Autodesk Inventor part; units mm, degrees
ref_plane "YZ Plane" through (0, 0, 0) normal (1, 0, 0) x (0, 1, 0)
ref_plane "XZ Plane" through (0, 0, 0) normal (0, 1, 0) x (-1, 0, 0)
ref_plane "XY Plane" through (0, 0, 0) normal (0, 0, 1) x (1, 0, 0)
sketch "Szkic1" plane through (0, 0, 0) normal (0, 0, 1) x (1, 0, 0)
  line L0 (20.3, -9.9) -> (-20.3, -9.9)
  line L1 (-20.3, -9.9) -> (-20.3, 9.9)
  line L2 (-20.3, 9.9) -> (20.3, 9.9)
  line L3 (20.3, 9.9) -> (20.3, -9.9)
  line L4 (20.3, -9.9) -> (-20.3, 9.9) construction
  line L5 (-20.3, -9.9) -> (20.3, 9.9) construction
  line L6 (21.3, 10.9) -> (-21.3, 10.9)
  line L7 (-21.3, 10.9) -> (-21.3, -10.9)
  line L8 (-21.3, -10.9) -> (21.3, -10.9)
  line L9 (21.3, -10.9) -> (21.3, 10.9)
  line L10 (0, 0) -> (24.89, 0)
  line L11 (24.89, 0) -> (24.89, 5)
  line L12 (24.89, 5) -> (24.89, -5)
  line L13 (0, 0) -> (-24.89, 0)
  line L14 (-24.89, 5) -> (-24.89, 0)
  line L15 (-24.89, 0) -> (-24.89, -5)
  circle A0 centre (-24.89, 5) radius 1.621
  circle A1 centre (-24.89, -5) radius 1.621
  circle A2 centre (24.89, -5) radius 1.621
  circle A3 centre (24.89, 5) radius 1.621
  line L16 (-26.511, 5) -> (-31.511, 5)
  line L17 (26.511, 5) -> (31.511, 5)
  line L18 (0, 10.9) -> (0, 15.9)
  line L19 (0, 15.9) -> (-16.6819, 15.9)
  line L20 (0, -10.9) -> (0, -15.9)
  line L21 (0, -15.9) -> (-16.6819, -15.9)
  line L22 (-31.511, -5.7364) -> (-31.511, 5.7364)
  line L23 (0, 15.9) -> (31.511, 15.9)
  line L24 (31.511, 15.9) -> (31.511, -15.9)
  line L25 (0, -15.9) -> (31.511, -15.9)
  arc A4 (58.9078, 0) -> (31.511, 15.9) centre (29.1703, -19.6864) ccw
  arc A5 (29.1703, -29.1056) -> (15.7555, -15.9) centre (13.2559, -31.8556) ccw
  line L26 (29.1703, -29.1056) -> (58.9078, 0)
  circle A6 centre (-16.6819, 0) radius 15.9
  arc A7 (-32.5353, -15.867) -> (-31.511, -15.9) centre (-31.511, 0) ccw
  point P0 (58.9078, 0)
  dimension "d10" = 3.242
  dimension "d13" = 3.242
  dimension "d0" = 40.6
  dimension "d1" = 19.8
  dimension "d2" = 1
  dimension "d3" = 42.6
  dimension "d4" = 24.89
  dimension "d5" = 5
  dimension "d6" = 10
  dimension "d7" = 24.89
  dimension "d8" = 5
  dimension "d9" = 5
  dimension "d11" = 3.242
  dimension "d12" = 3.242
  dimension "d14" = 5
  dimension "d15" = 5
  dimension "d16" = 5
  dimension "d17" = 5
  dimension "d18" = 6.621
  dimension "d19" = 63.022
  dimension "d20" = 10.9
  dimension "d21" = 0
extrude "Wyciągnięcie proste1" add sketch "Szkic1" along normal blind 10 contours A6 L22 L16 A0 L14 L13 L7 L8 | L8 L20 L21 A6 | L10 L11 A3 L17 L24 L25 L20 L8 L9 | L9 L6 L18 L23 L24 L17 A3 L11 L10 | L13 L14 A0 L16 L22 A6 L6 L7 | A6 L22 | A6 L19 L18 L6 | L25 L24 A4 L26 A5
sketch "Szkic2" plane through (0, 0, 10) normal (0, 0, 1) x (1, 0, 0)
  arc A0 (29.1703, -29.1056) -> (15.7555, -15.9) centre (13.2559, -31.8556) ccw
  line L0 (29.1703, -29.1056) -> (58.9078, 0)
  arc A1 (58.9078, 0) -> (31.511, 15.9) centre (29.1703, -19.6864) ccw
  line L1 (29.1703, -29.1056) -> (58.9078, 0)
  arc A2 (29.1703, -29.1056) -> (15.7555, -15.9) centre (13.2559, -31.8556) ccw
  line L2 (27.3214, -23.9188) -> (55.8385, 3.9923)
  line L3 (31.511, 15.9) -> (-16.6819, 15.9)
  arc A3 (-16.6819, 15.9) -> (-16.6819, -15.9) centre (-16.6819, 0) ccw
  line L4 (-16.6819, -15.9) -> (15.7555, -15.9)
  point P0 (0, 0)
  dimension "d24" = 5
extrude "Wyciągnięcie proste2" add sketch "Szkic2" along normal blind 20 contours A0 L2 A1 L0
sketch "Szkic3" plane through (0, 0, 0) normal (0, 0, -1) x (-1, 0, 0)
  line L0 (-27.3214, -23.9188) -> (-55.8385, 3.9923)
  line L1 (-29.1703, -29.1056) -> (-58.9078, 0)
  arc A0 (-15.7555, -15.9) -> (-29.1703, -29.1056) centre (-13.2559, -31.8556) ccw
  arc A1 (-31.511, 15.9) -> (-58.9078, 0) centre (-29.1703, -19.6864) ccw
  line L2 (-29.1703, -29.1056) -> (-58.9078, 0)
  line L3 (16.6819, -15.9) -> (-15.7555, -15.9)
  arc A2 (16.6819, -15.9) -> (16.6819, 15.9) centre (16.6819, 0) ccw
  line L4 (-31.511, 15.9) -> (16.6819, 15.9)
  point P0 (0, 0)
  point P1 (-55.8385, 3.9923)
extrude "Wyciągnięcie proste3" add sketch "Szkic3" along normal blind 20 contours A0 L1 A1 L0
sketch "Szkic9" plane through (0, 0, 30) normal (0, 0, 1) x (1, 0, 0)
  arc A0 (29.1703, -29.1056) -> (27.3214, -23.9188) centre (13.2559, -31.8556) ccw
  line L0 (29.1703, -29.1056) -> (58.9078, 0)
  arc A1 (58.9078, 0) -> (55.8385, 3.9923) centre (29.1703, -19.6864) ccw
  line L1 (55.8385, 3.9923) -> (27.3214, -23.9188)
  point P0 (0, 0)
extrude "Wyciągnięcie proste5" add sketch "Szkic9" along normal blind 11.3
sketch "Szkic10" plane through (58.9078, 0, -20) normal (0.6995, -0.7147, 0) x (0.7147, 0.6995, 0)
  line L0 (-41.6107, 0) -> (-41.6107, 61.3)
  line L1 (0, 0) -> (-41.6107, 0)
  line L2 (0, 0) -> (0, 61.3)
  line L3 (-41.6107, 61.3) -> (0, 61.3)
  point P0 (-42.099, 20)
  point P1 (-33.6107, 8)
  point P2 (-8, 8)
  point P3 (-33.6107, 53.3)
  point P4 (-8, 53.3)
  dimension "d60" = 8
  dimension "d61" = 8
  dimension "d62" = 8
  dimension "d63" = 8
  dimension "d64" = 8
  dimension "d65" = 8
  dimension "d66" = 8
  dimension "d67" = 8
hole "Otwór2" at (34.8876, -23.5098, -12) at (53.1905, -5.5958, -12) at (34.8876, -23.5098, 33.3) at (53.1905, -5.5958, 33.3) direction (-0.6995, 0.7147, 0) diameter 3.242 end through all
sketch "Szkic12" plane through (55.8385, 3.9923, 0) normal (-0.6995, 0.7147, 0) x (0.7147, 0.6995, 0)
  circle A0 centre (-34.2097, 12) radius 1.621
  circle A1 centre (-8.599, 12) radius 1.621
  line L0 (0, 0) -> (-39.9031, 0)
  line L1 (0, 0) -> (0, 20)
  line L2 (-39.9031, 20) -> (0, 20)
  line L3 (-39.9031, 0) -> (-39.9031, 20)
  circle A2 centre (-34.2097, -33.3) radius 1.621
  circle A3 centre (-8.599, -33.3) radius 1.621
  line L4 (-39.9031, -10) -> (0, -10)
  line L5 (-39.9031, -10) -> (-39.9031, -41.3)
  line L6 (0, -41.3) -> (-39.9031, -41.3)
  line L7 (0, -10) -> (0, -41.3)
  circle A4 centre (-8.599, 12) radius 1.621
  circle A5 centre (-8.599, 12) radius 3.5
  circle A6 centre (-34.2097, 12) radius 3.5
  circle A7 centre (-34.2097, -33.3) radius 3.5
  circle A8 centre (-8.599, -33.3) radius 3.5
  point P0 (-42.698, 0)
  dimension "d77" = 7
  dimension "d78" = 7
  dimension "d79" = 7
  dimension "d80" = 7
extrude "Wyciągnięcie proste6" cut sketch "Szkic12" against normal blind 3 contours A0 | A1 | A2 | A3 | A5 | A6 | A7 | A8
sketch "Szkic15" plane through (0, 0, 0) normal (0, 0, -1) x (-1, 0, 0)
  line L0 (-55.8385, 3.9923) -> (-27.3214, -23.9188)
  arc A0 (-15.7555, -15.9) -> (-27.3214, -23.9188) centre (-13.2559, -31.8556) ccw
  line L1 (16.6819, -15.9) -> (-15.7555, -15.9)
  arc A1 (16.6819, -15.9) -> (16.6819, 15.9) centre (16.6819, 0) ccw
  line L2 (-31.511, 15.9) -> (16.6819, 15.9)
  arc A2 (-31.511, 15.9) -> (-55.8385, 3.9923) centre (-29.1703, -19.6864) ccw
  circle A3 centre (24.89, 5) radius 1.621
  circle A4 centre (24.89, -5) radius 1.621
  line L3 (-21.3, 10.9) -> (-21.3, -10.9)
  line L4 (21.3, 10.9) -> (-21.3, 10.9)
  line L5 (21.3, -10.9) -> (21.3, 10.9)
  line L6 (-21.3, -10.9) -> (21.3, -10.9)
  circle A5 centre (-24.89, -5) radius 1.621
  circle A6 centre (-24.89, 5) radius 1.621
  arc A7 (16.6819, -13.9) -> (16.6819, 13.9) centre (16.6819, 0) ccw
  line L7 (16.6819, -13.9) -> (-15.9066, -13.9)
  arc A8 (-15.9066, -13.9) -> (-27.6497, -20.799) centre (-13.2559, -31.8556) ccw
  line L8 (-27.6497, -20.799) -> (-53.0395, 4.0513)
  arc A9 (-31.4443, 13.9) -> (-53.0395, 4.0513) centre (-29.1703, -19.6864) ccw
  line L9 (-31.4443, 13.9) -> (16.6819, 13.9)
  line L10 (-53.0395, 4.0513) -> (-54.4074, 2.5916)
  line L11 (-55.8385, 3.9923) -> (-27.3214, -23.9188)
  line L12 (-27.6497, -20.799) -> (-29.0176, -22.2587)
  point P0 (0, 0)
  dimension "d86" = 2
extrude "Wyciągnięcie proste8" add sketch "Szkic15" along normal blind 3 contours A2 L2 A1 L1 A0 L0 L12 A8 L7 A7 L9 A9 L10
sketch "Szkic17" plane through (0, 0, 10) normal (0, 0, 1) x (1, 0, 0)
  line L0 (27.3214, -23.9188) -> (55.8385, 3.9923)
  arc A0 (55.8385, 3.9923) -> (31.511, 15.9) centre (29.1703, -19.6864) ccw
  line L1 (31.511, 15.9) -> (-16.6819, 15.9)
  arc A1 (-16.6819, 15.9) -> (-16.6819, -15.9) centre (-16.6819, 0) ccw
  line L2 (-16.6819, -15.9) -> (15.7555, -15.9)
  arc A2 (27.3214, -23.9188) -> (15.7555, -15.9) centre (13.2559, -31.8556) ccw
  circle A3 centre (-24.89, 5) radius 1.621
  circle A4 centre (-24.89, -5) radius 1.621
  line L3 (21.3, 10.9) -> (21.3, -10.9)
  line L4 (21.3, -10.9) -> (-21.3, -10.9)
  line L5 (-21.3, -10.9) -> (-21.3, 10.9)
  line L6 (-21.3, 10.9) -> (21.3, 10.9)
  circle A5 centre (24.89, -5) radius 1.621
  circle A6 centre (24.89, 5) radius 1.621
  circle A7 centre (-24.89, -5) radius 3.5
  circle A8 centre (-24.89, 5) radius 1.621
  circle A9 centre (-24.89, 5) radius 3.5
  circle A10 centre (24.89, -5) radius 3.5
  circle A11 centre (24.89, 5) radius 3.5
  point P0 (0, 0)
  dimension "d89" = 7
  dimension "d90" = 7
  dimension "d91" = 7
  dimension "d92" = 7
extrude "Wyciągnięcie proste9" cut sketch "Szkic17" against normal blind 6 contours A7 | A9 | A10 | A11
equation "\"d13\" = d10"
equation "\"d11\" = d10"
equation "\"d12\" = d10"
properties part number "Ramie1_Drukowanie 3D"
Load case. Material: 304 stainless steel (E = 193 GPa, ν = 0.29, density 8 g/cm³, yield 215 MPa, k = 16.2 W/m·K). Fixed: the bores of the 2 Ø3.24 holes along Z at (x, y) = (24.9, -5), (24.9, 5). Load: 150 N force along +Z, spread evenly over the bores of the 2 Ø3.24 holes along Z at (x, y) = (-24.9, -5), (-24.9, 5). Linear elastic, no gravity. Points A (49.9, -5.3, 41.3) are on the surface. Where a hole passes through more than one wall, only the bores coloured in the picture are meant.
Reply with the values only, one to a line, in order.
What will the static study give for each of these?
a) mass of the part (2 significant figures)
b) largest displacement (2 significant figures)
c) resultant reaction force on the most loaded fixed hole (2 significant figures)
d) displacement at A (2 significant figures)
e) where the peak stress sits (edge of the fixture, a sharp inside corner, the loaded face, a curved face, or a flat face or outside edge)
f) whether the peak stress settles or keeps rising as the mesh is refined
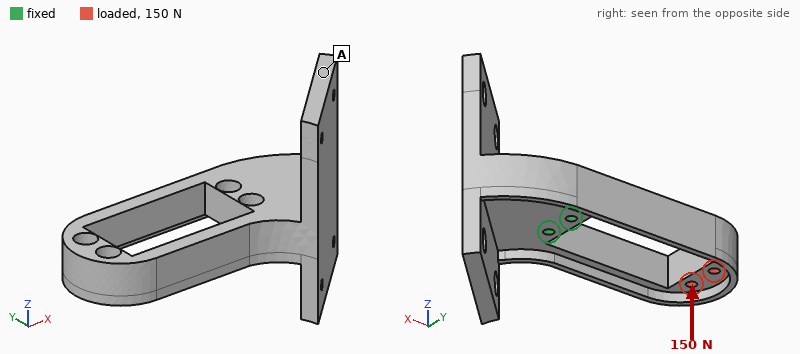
220 g
73 µm
100 N
28 µm
edge of the fixture
keeps rising
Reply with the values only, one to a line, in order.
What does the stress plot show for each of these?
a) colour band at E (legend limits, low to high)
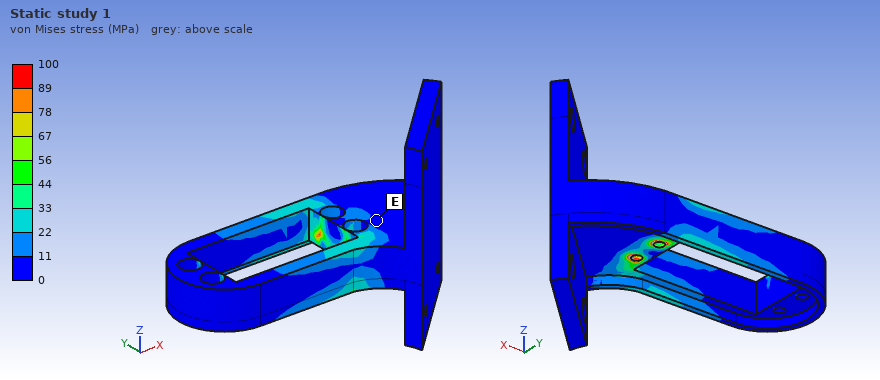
0 to 11 MPa
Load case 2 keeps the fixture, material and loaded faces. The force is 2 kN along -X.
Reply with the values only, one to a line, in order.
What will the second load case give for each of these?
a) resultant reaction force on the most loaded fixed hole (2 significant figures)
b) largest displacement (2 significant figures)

1.0 kN
45 µm
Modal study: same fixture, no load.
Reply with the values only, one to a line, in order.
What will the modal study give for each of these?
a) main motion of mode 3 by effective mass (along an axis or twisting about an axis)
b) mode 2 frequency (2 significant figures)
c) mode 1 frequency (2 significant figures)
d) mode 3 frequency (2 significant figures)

along Z
1700 Hz
1200 Hz
2500 Hz
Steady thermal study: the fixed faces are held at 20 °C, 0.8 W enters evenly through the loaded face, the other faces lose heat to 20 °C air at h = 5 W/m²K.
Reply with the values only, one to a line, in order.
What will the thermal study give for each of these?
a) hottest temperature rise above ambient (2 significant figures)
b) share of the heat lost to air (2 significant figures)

21 K
41 %
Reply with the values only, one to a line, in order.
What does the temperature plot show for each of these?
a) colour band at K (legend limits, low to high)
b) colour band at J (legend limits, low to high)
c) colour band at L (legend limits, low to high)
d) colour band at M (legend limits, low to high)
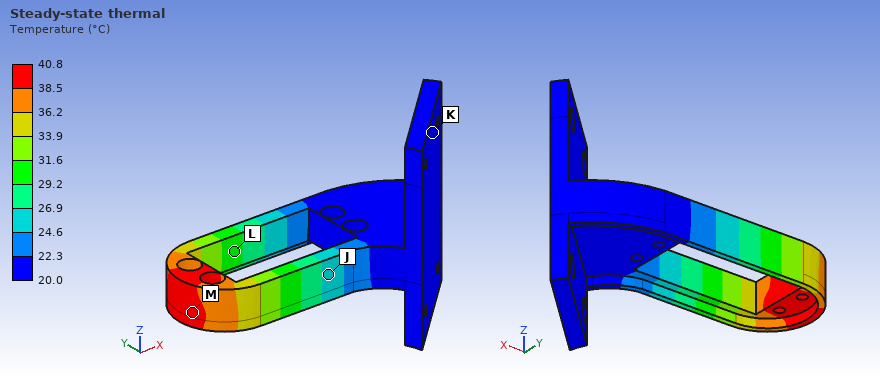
20.0 to 22.3 °C
24.6 to 26.9 °C
29.2 to 31.6 °C
38.5 to 40.8 °C
